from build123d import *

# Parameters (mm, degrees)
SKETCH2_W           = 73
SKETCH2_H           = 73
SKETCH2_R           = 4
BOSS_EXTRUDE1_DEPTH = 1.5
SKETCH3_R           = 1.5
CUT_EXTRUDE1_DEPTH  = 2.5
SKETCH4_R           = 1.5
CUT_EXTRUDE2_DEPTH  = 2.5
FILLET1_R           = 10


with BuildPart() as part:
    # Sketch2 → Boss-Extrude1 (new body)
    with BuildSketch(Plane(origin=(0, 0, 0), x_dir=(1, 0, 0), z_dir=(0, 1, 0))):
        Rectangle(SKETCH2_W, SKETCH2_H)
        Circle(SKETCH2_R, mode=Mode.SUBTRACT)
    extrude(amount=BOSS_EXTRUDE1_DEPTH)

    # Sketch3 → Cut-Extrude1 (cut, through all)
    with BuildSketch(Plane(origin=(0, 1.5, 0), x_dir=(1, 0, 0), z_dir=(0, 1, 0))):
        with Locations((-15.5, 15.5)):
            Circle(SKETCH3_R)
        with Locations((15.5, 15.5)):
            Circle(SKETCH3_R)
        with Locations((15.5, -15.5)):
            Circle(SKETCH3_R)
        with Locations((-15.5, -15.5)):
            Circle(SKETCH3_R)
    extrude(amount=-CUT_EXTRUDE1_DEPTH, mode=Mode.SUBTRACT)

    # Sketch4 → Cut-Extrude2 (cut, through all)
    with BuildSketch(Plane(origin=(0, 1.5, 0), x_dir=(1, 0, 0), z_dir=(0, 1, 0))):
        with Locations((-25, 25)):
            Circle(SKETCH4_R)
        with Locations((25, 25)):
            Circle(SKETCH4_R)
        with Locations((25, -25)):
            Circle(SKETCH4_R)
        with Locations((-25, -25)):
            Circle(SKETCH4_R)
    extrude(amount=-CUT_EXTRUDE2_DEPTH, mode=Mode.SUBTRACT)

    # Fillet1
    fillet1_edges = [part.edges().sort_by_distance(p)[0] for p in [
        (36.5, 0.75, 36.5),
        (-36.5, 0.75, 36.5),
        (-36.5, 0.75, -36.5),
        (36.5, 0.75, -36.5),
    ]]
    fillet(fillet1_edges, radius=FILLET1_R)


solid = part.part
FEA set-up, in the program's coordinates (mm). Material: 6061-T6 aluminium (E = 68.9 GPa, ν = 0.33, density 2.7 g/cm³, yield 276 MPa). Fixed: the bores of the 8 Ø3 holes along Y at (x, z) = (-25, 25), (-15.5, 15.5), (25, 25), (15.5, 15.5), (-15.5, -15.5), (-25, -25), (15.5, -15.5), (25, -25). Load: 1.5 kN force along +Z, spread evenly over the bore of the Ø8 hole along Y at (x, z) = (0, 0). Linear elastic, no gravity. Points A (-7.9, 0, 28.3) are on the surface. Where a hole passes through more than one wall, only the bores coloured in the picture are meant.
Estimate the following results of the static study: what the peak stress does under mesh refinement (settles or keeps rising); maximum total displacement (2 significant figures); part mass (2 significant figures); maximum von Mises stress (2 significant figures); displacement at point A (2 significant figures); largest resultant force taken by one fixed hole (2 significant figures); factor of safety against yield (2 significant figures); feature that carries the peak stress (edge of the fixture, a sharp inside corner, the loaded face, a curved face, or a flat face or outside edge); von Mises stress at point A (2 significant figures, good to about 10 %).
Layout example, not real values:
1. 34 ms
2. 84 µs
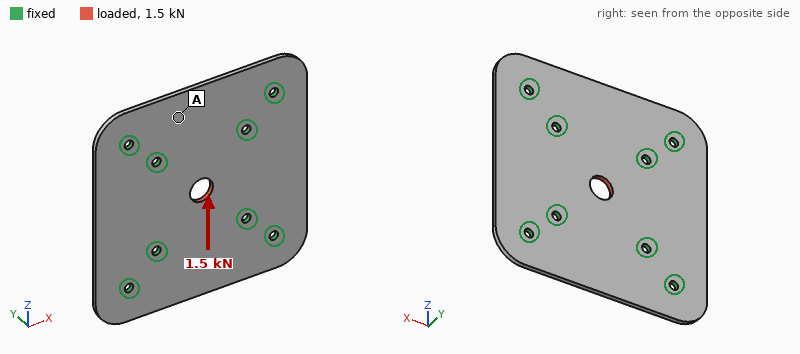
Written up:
1. settles
2. 8.3 µm
3. 21 g
4. 70 MPa
5. 2.3 µm
6. 330 N
7. 3.9
8. the loaded face
9. 6.1 MPa
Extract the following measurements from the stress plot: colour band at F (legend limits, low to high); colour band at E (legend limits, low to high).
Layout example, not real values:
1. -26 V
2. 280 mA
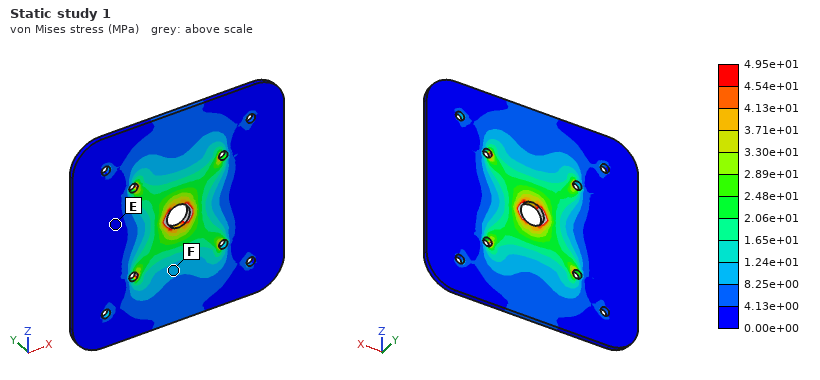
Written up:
1. 8.25e+00 to 1.24e+01 MPa
2. 0.00e+00 to 4.13e+00 MPa
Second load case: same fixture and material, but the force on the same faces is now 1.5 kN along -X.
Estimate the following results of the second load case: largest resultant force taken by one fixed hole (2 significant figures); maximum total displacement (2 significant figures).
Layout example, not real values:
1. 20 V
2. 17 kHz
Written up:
1. 330 N
2. 8.3 µm
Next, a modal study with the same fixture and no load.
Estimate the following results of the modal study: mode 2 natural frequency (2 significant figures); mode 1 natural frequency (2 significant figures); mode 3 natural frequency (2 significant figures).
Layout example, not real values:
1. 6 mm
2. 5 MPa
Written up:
1. 4000 Hz
2. 3800 Hz
3. 4000 Hz
